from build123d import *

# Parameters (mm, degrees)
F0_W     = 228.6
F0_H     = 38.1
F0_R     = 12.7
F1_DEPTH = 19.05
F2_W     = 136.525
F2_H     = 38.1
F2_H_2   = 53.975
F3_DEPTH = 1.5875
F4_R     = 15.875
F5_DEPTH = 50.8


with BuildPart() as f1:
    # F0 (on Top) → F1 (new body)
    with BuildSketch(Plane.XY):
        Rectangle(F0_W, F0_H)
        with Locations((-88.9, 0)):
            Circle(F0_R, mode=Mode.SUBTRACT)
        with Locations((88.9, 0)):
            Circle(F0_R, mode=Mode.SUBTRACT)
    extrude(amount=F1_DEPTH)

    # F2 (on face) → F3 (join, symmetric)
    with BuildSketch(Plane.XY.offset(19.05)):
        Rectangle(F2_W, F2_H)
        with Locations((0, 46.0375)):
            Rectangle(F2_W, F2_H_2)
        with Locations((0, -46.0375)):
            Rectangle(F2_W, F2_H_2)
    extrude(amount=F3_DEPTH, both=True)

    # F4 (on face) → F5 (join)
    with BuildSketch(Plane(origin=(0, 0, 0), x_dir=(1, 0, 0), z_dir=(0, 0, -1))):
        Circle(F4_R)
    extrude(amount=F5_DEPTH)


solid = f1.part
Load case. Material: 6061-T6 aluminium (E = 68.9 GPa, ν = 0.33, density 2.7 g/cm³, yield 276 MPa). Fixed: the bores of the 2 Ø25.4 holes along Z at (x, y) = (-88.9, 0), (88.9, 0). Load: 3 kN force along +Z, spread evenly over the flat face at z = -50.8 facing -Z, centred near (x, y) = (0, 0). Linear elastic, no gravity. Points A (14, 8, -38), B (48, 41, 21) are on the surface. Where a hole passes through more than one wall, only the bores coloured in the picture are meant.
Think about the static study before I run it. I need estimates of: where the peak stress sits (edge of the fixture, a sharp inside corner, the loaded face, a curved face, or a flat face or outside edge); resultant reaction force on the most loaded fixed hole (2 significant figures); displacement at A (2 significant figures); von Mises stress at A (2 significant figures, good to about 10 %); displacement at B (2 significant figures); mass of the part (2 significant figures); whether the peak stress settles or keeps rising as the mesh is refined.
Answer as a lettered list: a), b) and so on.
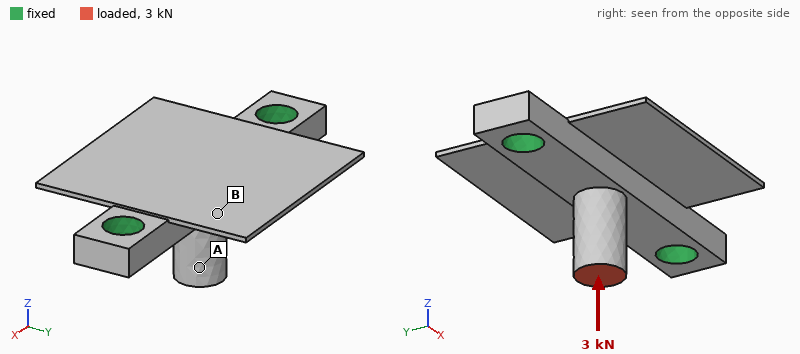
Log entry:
a) edge of the fixture
b) 1.5 kN
c) 33 µm
d) 3.8 MPa
e) 15 µm
f) 650 g
g) keeps rising
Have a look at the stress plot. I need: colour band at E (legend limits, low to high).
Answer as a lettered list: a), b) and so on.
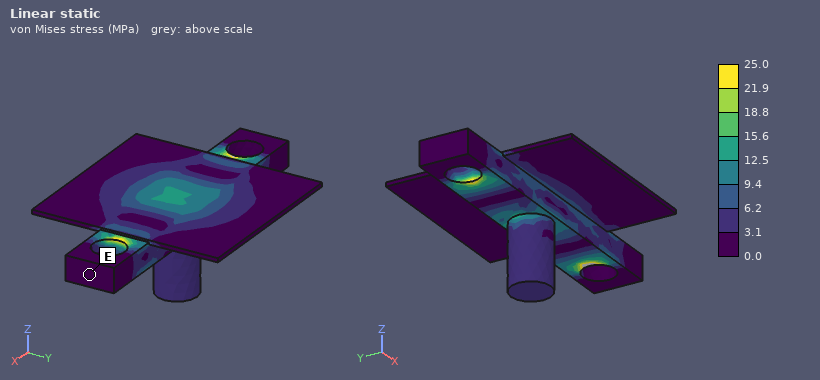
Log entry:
a) 0.0 to 3.1 MPa
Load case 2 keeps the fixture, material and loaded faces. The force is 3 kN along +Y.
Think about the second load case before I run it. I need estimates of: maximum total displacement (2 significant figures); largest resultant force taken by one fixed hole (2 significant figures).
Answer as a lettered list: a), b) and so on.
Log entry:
a) 0.28 mm
b) 1.5 kN
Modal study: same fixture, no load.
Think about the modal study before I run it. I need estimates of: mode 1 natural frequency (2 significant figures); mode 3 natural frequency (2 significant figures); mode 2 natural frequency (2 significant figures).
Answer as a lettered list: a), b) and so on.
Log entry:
a) 880 Hz
b) 1200 Hz
c) 910 Hz
